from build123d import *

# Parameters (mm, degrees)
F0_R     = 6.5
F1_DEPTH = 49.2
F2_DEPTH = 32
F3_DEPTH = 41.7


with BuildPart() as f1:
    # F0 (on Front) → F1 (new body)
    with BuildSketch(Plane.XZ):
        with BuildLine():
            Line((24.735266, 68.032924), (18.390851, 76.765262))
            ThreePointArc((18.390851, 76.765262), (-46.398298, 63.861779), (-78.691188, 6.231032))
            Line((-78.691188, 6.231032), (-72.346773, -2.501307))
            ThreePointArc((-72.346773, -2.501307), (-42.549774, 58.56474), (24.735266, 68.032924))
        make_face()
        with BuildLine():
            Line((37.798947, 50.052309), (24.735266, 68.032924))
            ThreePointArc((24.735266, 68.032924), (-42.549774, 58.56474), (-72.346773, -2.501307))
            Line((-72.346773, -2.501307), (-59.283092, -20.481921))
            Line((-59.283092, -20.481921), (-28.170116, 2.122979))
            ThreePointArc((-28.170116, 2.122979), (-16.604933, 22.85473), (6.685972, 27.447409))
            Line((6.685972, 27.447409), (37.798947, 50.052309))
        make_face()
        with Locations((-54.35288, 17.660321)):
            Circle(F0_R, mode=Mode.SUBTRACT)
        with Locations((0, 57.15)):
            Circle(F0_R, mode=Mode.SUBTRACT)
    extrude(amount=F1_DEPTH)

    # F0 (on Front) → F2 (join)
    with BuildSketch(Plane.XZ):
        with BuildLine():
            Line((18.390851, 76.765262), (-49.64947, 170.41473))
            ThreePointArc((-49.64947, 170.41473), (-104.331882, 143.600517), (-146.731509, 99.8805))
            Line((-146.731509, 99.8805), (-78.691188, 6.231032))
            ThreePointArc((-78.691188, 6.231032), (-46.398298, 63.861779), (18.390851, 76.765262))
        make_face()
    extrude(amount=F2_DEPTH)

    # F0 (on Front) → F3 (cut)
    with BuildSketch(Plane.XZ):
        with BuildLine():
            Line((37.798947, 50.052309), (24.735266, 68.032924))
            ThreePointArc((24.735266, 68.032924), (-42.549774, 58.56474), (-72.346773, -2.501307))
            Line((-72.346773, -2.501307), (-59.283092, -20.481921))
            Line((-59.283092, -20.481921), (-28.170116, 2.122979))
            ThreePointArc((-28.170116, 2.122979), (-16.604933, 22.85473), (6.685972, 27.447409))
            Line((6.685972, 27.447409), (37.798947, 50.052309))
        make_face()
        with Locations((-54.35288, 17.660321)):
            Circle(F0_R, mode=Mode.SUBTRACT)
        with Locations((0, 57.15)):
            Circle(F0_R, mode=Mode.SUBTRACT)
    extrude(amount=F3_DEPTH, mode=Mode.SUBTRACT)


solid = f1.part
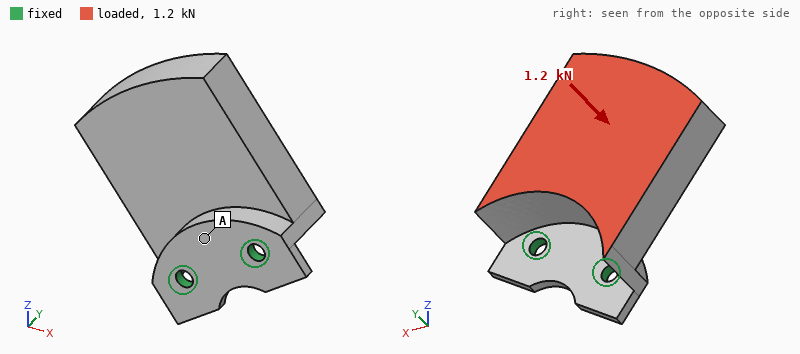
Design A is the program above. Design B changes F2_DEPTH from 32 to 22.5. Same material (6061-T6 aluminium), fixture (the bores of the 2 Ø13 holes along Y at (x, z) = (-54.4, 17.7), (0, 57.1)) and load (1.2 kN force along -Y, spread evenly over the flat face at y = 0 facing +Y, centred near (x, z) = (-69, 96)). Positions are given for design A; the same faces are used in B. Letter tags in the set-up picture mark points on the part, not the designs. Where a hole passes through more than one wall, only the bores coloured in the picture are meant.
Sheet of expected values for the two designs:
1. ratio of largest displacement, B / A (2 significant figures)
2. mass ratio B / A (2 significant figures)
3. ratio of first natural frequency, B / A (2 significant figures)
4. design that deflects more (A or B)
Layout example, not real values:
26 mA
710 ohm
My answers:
1.1
0.75
1.1
B
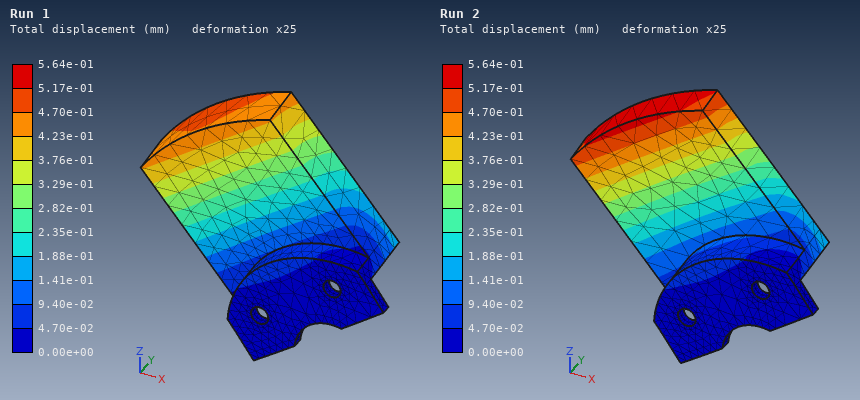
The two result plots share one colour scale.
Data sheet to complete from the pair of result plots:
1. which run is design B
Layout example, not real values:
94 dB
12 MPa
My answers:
Run 2
